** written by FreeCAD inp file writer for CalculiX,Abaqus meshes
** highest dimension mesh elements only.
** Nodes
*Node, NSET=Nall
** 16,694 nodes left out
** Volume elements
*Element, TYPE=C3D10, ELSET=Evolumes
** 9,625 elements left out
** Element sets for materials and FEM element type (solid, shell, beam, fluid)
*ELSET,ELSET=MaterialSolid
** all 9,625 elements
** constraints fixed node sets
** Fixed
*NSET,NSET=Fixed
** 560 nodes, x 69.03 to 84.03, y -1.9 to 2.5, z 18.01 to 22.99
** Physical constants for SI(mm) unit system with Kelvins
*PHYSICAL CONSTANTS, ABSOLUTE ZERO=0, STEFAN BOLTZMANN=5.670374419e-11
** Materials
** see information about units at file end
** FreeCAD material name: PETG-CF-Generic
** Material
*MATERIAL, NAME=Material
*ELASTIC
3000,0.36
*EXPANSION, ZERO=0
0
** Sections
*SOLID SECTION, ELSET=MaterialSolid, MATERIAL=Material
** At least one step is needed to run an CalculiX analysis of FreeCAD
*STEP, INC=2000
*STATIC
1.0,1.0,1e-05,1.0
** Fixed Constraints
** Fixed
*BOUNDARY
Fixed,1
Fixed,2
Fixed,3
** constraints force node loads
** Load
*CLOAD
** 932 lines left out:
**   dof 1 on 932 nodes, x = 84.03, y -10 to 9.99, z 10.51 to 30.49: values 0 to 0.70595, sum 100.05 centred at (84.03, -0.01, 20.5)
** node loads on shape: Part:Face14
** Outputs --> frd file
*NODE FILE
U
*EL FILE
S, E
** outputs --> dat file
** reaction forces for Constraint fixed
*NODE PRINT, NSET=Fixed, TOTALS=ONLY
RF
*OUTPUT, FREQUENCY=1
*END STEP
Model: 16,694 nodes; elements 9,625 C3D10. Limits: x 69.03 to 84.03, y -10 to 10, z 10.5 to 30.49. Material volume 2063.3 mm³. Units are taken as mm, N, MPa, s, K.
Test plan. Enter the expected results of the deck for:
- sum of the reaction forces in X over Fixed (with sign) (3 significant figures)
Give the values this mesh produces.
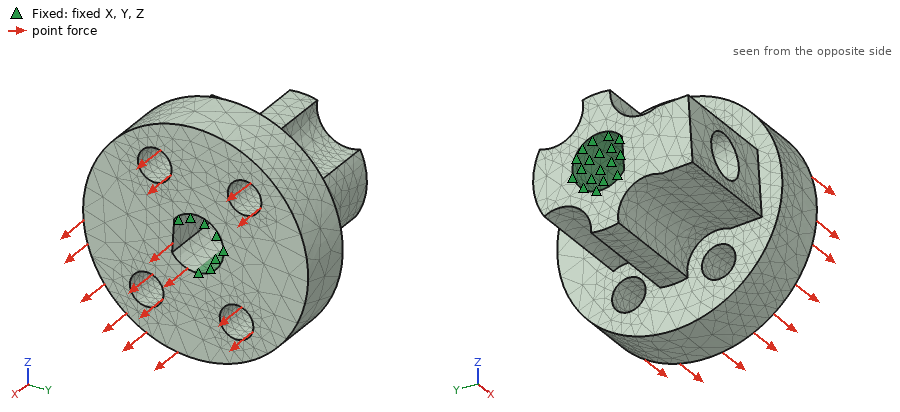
-100 N
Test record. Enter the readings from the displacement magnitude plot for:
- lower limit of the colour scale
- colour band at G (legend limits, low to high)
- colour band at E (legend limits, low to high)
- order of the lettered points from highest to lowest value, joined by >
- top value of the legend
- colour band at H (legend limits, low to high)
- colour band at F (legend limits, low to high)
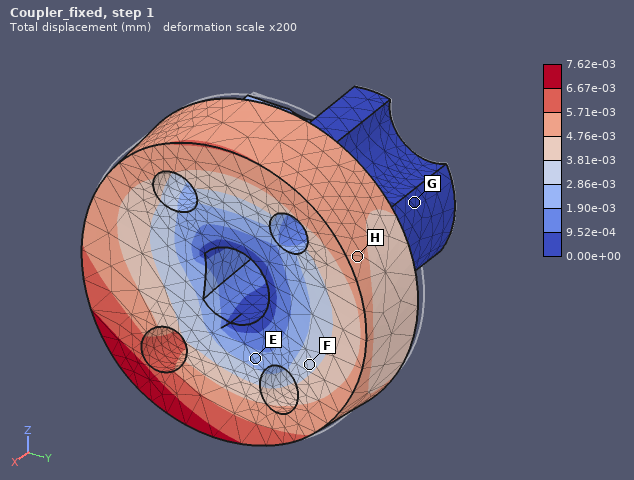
0.00e+00 mm
0.00e+00 to 9.52e-04 mm
1.90e-03 to 2.86e-03 mm
H > F > E > G
7.62e-03 mm
4.76e-03 to 5.71e-03 mm
2.86e-03 to 3.81e-03 mm
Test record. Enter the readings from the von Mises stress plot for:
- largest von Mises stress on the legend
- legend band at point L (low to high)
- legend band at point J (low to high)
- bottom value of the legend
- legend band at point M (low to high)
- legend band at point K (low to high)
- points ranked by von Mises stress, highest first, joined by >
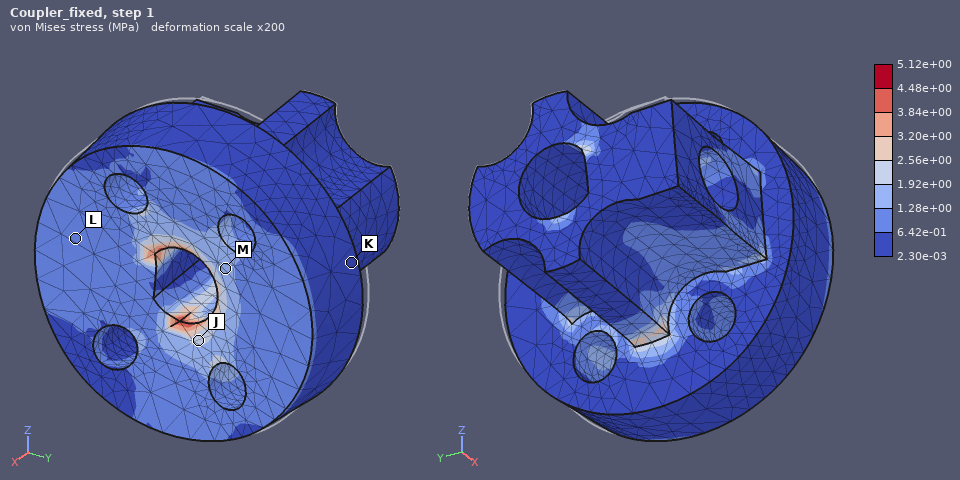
5.12e+00 MPa
6.42e-01 to 1.28e+00 MPa
1.92e+00 to 2.56e+00 MPa
2.30e-03 MPa
1.28e+00 to 1.92e+00 MPa
2.30e-03 to 6.42e-01 MPa
J > M > L > K
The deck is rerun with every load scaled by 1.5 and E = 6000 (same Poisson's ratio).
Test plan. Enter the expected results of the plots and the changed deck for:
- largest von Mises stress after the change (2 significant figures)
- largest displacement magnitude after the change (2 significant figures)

7.7 MPa
0.0057 mm
